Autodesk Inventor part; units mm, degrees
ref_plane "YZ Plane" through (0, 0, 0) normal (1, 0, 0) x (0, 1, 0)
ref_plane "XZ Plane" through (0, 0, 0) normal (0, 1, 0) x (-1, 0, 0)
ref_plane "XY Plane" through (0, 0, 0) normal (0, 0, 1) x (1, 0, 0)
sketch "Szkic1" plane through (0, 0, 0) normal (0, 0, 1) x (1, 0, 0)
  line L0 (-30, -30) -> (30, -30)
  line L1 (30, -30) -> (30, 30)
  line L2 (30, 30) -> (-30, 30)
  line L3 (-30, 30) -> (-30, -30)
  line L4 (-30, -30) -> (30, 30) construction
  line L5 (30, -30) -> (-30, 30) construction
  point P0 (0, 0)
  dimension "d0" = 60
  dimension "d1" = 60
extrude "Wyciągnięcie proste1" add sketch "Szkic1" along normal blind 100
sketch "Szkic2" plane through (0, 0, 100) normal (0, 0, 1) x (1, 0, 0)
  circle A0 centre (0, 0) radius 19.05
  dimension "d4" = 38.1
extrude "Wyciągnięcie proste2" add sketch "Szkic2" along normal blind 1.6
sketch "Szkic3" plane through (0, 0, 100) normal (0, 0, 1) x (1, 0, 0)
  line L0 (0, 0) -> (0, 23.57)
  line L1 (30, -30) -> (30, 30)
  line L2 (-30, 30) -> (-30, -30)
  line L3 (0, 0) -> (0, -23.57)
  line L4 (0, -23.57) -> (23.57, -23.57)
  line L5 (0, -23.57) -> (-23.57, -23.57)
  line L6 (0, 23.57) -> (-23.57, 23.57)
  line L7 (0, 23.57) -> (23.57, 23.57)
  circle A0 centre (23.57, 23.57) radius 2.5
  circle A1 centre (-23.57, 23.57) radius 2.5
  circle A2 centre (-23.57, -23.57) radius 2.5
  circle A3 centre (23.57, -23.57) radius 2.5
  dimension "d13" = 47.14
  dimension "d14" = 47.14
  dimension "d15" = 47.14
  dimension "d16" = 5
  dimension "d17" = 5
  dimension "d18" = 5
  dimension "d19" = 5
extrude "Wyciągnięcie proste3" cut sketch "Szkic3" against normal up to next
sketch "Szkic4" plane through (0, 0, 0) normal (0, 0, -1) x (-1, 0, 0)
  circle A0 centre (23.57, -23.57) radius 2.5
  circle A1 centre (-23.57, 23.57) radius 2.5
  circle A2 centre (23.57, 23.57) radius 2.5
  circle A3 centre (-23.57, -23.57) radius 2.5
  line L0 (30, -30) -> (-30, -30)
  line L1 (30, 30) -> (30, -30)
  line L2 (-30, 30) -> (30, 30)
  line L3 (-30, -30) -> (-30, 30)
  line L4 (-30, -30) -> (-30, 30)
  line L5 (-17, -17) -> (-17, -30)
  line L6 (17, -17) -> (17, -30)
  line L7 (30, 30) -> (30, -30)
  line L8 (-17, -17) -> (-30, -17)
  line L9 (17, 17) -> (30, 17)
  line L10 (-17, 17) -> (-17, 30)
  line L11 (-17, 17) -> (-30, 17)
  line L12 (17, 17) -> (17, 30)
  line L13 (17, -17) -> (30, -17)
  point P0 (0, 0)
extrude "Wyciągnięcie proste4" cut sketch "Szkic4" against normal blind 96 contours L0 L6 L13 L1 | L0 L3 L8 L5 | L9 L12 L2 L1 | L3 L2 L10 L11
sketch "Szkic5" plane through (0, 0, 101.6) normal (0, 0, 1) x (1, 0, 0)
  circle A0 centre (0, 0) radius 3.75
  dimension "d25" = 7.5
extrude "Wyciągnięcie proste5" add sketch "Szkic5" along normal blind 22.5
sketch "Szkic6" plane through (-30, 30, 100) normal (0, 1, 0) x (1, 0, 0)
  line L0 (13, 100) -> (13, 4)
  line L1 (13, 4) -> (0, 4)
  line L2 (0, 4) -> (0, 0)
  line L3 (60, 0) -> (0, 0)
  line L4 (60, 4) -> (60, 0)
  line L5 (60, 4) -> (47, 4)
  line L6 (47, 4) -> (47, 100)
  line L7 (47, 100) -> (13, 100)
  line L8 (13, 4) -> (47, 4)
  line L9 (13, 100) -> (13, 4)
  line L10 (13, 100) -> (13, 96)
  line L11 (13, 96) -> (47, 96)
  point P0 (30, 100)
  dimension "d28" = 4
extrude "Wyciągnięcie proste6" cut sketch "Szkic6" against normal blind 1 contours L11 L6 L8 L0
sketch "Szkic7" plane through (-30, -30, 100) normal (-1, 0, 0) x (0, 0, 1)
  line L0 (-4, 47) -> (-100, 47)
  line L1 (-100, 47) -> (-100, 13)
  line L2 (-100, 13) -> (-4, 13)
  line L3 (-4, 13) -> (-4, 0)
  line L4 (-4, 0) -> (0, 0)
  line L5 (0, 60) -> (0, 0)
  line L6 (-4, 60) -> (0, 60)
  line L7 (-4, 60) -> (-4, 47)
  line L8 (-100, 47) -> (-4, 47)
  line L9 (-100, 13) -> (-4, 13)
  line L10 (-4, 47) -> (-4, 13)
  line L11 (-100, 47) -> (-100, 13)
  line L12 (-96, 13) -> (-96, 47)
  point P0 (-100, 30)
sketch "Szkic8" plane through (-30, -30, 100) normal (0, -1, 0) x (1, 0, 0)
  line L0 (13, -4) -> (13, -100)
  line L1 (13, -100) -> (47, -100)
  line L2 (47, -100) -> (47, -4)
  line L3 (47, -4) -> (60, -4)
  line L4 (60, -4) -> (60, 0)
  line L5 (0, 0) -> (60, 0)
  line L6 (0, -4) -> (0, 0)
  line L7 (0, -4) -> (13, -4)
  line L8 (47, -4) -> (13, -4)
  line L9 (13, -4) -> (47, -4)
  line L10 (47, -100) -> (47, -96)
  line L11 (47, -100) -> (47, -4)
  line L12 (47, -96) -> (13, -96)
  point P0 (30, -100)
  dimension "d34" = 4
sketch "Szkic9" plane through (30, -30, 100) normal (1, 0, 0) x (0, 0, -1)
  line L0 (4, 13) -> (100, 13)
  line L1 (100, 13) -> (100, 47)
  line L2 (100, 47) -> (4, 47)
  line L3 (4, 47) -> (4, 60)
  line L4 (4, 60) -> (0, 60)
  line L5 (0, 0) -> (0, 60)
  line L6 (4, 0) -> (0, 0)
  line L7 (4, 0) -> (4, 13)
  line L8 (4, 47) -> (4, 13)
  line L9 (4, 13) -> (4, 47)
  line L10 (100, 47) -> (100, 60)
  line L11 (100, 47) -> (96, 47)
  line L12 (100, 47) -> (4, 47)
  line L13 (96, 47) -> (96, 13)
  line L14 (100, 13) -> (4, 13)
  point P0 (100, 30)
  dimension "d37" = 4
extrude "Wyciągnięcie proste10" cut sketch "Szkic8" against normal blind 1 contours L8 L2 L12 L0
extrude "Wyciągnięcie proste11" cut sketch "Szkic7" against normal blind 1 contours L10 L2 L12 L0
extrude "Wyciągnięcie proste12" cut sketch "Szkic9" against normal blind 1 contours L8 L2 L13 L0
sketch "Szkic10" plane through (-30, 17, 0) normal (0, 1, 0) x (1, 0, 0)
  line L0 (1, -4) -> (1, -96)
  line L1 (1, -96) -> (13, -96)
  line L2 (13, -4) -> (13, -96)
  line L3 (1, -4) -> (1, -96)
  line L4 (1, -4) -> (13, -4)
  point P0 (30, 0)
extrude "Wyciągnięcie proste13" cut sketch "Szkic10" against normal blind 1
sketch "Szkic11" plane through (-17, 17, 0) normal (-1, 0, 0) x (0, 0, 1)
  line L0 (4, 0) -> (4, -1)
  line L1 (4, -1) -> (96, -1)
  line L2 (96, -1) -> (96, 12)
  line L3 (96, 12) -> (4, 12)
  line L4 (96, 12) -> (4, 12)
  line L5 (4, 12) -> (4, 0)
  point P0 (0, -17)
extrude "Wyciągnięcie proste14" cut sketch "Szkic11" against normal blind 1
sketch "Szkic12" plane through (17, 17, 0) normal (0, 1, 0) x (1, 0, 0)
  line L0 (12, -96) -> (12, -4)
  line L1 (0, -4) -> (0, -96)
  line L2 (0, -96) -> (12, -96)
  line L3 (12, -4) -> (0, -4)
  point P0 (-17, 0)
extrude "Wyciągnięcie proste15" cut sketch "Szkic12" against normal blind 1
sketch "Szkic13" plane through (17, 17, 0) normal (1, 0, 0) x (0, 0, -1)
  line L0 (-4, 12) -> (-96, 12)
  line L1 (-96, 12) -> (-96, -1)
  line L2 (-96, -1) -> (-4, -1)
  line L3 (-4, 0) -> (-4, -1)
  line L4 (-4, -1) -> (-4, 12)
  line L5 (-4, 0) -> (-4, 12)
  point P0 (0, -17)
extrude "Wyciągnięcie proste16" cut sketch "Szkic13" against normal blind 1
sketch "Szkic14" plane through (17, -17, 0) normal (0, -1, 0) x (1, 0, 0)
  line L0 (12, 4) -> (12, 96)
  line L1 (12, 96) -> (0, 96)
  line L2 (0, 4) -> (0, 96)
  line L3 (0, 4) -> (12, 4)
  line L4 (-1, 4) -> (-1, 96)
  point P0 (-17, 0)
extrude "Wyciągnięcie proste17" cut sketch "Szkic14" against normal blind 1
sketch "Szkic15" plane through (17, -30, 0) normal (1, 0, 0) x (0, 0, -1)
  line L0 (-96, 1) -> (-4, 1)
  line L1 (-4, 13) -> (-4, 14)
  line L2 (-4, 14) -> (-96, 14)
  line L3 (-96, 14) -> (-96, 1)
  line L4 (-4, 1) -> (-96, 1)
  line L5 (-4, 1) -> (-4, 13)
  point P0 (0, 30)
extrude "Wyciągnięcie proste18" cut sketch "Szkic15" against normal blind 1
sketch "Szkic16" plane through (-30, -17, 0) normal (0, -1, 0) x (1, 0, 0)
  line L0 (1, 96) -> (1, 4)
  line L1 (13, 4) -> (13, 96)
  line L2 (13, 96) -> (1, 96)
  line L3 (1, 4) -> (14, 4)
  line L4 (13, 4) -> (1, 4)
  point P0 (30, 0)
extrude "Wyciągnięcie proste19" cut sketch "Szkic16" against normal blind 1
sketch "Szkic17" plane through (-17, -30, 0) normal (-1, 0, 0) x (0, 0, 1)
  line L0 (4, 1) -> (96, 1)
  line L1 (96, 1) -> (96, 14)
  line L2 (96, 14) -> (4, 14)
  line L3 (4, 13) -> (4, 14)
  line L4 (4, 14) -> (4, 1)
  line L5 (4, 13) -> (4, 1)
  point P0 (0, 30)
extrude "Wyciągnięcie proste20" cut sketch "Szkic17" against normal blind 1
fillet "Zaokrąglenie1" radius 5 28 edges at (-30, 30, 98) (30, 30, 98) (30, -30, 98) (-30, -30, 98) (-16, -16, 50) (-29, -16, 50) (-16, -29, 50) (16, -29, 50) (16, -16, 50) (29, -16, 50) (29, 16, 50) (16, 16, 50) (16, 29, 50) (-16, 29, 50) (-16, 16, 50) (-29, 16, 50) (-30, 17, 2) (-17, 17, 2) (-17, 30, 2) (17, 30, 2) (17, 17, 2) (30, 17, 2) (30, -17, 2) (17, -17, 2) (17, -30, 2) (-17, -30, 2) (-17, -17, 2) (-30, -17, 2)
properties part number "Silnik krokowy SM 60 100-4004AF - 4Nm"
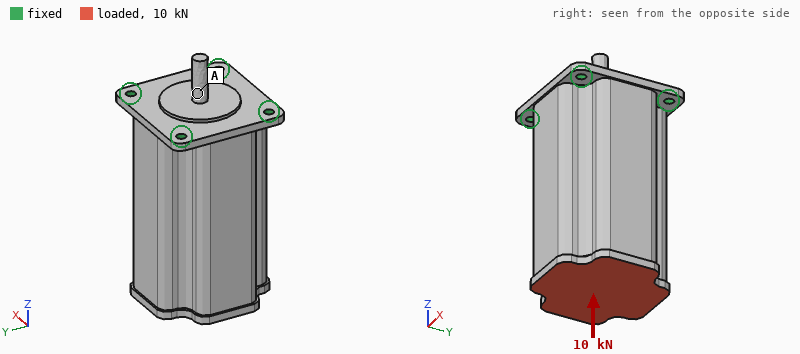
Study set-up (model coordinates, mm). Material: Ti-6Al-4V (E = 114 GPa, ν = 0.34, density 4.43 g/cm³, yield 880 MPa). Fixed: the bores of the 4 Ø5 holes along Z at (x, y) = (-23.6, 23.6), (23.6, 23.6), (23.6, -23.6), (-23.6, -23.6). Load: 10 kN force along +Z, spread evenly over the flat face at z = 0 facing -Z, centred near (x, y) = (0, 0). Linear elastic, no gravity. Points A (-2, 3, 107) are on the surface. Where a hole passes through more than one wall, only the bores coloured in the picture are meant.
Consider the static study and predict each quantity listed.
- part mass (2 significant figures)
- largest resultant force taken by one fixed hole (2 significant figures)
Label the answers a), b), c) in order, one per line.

a) 1.2 kg
b) 2.7 kN
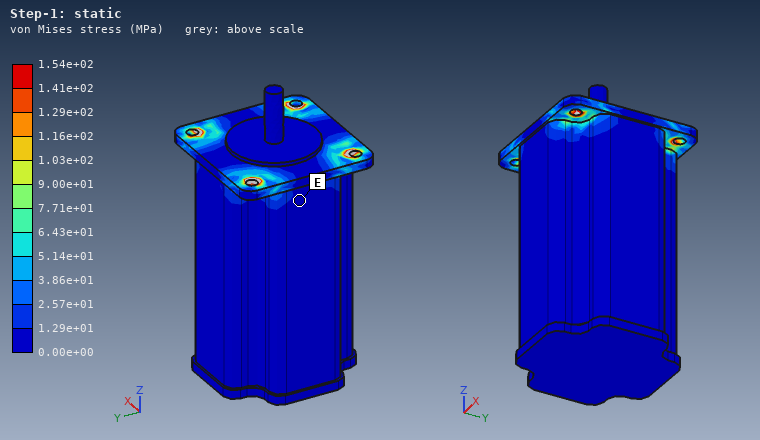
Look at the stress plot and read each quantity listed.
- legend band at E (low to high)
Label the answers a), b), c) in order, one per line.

a) 0.00e+00 to 1.29e+01 MPa
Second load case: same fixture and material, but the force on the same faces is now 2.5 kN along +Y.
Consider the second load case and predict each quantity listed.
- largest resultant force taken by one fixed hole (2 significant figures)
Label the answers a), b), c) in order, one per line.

a) 3.0 kN
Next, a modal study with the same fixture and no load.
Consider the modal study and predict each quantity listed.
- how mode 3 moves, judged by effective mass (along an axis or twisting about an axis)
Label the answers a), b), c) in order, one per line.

a) along Z
